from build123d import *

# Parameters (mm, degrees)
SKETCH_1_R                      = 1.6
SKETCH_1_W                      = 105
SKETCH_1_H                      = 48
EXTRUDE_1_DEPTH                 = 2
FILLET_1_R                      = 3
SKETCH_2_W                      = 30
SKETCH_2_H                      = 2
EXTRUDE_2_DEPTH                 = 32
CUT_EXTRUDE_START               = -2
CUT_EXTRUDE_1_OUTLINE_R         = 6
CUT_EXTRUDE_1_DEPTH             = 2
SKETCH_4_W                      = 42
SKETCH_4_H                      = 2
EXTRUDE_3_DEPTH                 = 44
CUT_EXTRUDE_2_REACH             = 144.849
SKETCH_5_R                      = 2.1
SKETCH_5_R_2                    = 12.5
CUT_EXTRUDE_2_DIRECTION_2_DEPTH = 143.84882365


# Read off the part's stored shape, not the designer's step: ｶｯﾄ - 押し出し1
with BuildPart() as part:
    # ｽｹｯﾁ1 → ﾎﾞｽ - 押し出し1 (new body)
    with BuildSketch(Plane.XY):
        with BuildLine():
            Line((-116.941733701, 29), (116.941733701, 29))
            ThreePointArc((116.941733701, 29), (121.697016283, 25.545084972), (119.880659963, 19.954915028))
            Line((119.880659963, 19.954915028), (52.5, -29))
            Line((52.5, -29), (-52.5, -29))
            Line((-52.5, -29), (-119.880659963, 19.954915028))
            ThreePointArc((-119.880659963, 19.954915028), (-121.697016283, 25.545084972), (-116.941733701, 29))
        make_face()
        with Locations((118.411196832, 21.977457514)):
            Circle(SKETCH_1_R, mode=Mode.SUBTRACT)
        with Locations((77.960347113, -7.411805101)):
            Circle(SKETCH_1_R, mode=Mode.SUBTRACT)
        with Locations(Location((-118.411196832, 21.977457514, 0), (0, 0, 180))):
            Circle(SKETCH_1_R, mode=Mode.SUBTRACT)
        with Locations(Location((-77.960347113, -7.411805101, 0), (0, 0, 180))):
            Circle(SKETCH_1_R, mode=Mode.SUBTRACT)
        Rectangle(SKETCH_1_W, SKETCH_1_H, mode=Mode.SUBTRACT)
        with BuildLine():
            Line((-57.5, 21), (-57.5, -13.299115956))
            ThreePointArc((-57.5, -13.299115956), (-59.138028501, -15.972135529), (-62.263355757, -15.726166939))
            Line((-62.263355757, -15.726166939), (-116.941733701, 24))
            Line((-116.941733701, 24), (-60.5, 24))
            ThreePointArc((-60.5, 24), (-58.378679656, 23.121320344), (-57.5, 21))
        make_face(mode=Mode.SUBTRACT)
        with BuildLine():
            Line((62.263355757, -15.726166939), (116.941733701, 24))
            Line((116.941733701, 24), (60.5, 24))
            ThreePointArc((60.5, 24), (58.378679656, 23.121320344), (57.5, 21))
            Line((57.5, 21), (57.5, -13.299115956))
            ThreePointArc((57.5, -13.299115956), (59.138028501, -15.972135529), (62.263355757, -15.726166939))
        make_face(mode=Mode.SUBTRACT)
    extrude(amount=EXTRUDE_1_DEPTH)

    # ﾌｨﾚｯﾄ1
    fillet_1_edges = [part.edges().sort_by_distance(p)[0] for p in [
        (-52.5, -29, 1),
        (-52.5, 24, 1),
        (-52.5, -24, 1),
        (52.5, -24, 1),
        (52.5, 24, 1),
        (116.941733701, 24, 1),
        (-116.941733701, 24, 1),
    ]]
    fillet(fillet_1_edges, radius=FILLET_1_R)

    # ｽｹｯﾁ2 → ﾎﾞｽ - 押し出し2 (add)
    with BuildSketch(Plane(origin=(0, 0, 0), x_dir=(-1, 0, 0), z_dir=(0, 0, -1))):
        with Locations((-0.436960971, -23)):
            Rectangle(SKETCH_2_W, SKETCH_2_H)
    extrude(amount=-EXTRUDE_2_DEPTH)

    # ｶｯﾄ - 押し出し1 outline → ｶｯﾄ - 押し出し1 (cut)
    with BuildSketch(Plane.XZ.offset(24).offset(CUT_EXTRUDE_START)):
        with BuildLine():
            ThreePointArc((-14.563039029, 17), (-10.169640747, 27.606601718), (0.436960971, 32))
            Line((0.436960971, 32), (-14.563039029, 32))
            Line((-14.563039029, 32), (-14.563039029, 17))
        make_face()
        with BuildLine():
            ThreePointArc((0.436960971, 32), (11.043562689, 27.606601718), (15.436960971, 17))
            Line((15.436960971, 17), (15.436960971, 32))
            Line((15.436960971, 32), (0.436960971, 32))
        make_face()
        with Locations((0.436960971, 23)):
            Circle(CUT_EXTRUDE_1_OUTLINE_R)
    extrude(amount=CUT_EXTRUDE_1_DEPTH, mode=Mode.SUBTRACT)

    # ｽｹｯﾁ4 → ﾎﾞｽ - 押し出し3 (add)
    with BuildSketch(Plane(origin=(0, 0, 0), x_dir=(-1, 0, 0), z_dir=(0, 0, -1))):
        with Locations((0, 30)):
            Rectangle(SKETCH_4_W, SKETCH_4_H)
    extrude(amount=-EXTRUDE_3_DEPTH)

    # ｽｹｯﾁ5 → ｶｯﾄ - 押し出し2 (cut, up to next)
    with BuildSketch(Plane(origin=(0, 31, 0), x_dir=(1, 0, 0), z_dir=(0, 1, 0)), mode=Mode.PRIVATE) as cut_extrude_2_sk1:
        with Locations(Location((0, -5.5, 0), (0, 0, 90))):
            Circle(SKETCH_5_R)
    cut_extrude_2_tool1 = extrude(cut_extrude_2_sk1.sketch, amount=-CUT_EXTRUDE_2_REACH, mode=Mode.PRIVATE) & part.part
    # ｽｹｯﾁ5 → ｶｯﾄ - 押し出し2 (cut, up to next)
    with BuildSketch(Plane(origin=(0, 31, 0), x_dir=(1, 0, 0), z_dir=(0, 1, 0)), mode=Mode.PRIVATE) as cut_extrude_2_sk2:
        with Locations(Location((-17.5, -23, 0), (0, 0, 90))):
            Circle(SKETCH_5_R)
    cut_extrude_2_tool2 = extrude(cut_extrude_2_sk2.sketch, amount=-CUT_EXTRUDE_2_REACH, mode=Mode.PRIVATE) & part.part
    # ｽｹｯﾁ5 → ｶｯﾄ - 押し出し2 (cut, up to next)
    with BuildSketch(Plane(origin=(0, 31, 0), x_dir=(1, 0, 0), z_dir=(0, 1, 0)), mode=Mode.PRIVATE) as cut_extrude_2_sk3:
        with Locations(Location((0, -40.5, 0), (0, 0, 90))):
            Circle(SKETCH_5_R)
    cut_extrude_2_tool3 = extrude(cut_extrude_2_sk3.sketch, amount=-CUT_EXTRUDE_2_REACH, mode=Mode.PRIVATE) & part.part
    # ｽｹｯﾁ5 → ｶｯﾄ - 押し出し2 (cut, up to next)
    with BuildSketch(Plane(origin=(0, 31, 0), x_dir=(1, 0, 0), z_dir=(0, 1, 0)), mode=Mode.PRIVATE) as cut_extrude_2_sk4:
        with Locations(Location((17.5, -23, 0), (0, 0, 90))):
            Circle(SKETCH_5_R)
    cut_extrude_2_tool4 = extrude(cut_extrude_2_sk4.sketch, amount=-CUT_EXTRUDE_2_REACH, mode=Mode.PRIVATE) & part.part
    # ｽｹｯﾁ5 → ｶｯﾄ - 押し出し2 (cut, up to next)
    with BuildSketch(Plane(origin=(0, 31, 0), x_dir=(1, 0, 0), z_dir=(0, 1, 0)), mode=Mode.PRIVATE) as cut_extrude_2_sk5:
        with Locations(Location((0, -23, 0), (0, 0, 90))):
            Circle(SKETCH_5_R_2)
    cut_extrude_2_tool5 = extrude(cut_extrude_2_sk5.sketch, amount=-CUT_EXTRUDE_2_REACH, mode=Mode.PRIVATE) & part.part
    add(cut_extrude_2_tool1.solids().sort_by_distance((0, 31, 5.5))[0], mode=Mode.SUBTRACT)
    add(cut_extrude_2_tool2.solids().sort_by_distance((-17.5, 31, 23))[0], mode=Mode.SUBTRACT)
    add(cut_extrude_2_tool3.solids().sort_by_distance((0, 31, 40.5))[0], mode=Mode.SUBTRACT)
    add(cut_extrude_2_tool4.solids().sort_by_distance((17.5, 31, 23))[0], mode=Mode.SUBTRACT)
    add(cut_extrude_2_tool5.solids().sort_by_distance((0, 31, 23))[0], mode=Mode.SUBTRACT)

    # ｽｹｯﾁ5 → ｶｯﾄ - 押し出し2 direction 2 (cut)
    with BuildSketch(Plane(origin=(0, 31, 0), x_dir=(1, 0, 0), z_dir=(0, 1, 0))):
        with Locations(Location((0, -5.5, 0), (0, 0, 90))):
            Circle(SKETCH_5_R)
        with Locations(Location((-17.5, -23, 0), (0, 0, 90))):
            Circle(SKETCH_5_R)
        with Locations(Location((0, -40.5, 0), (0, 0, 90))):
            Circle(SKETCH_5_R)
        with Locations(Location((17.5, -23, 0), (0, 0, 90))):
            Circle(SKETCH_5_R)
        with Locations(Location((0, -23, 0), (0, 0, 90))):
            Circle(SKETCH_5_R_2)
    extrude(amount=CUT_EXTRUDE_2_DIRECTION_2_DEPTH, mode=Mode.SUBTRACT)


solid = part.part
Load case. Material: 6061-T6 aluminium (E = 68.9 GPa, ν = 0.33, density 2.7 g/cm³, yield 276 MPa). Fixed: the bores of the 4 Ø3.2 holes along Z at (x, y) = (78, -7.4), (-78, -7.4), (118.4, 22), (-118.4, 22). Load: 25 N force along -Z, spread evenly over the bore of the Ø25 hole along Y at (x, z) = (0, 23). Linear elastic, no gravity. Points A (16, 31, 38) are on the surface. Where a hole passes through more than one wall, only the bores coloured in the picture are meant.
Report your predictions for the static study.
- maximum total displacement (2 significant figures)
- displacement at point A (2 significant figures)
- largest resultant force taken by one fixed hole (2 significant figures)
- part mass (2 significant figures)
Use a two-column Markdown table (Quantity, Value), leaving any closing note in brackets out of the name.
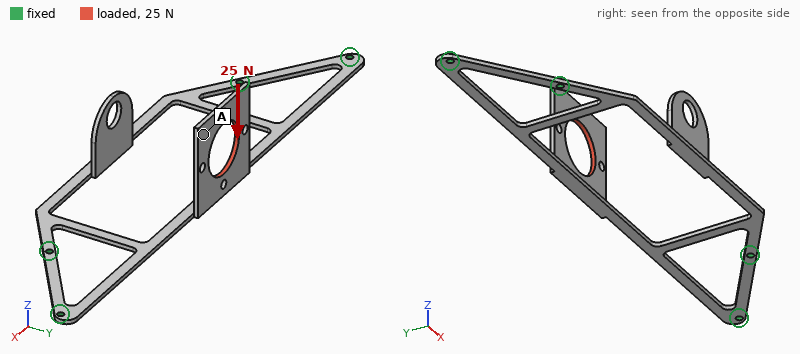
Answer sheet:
| Quantity | Value |
|---|---|
| maximum total displacement | 2.7 mm |
| displacement at point A | 2.6 mm |
| largest resultant force taken by one fixed hole | 6.9 N |
| part mass | 28 g |
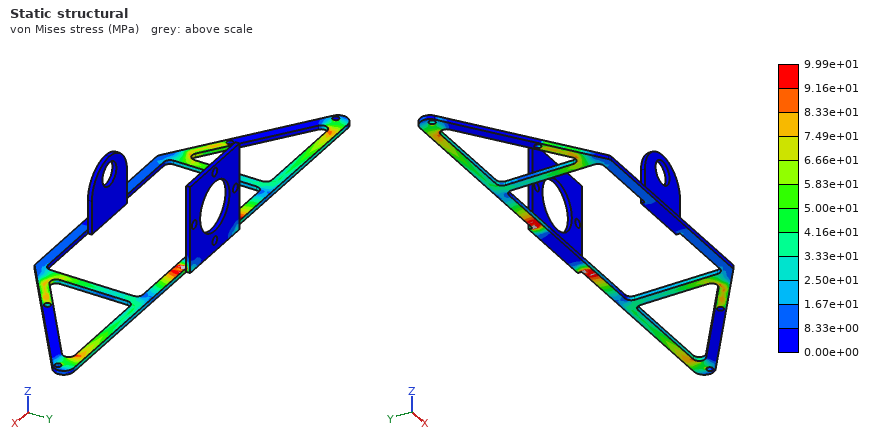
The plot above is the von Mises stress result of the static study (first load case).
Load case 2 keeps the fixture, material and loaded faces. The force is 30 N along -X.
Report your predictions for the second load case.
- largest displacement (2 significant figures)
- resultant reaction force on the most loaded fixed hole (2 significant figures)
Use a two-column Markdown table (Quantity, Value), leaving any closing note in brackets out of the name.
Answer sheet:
| Quantity | Value |
|---|---|
| largest displacement | 0.72 mm |
| resultant reaction force on the most loaded fixed hole | 14 N |
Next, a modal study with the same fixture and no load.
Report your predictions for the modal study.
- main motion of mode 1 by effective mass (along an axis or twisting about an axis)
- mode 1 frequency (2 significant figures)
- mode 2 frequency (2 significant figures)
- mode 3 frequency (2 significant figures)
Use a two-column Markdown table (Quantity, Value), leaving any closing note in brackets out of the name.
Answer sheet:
| Quantity | Value |
|---|---|
| main motion of mode 1 by effective mass | along Z |
| mode 1 frequency | 160 Hz |
| mode 2 frequency | 250 Hz |
| mode 3 frequency | 300 Hz |
